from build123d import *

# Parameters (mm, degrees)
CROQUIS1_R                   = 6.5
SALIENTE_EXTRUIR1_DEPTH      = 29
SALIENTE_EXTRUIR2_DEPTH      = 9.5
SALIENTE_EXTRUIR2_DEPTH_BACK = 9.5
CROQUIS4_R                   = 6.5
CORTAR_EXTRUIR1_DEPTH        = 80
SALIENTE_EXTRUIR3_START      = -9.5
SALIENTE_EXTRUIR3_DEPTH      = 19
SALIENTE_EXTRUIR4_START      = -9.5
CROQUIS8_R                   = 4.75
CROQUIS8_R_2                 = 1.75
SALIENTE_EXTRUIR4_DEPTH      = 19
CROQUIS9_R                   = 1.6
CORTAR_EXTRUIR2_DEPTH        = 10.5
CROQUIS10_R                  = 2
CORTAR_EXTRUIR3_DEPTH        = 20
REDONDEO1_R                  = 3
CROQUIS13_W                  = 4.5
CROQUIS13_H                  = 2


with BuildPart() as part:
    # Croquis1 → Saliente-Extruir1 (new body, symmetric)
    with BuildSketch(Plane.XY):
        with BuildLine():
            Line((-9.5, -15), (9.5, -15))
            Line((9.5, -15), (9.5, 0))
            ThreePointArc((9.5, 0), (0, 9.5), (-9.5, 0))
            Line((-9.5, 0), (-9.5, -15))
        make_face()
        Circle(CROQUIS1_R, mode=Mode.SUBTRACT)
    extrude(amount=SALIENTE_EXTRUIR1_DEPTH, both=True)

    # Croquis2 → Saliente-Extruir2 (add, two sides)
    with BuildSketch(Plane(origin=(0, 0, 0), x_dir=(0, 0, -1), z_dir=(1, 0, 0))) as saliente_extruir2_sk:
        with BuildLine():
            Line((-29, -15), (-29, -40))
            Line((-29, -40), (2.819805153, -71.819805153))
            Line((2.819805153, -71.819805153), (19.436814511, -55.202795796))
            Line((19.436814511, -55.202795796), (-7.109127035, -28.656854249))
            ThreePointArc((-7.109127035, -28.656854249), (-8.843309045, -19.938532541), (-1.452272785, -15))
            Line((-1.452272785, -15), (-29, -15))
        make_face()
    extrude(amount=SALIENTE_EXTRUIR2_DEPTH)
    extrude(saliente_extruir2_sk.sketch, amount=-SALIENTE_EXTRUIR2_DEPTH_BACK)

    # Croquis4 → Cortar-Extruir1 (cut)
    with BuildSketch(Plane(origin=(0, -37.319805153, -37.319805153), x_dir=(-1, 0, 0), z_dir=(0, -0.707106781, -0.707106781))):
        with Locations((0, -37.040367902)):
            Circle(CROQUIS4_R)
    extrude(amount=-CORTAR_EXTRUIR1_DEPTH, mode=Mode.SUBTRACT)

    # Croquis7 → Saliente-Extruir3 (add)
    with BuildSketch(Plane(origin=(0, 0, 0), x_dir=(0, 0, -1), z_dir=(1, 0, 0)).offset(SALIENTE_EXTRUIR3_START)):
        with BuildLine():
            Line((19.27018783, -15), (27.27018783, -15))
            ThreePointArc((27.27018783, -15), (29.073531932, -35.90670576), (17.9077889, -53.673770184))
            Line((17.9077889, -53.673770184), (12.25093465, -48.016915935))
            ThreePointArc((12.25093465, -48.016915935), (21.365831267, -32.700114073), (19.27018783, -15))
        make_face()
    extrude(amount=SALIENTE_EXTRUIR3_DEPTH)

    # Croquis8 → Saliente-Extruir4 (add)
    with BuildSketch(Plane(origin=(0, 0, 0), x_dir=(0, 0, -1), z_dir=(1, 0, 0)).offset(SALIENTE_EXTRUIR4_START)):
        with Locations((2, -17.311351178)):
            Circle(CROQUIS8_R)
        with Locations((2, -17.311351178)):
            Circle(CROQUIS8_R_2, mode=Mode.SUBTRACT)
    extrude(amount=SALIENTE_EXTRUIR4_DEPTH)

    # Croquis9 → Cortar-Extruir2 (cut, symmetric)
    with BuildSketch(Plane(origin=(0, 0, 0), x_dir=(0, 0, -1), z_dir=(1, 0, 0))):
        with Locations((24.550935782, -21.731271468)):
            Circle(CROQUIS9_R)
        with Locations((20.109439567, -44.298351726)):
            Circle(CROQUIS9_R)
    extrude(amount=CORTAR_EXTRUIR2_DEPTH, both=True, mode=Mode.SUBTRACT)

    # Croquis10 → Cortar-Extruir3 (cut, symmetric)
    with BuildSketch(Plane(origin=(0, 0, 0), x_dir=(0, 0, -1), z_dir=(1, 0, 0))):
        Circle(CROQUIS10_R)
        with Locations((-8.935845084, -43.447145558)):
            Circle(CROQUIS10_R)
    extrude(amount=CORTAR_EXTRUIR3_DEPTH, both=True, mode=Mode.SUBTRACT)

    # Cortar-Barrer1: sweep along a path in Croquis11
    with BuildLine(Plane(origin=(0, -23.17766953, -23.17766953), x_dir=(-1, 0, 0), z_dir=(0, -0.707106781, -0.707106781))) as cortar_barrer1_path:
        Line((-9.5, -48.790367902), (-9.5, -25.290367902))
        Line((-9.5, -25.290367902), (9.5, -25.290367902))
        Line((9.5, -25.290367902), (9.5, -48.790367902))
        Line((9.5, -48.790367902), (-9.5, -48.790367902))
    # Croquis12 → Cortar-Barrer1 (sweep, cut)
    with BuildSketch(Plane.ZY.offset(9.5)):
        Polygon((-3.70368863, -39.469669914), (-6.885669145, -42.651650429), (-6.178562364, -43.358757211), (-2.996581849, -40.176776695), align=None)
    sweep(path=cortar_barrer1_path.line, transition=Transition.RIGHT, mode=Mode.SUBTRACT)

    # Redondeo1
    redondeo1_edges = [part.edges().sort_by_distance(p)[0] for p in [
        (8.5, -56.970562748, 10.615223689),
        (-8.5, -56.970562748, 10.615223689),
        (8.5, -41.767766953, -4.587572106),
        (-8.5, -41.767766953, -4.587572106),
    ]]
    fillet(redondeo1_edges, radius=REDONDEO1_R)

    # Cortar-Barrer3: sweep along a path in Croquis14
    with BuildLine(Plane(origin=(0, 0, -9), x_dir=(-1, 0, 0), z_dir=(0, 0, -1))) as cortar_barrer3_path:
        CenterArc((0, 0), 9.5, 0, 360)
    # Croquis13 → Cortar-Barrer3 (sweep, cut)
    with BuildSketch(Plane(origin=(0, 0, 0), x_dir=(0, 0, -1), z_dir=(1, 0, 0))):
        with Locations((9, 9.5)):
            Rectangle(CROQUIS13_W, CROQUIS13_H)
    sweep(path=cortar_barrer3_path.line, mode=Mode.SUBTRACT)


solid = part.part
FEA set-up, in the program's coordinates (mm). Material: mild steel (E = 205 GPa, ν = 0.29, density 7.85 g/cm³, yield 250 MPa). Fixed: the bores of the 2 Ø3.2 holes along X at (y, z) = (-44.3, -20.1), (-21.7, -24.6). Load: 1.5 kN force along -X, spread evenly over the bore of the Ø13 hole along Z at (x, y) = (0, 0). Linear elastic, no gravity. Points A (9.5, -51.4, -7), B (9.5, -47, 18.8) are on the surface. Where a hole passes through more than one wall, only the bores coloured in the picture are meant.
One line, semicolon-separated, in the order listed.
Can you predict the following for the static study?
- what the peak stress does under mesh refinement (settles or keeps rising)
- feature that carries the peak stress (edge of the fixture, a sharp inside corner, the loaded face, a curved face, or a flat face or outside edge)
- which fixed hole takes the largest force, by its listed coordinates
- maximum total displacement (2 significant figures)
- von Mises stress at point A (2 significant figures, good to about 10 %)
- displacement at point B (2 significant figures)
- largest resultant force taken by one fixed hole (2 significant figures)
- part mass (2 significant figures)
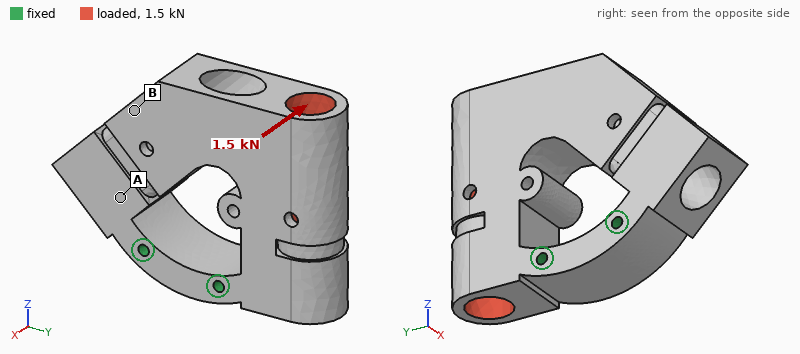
keeps rising; edge of the fixture; (-21.7, -24.6); 50 µm; 16 MPa; 18 µm; 1.4 kN; 330 g
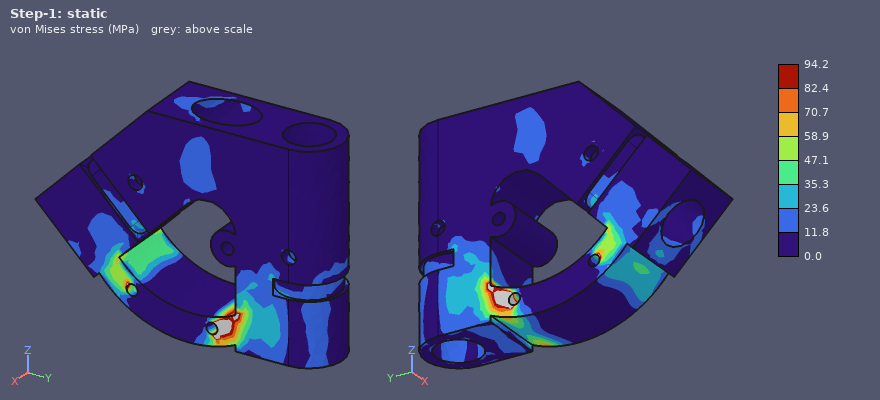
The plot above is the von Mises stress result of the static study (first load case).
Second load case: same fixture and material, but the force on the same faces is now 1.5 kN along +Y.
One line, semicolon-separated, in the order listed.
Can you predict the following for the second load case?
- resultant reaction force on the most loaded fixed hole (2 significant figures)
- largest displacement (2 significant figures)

1.2 kN; 15 µm
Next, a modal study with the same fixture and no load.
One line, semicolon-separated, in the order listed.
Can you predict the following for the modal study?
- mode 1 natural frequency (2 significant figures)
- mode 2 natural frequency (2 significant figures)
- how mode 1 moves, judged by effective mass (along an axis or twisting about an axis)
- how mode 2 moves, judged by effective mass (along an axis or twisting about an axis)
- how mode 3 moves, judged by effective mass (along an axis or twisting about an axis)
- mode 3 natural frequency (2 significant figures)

2400 Hz; 3200 Hz; along X; along Y; twisting about Z; 6100 Hz
